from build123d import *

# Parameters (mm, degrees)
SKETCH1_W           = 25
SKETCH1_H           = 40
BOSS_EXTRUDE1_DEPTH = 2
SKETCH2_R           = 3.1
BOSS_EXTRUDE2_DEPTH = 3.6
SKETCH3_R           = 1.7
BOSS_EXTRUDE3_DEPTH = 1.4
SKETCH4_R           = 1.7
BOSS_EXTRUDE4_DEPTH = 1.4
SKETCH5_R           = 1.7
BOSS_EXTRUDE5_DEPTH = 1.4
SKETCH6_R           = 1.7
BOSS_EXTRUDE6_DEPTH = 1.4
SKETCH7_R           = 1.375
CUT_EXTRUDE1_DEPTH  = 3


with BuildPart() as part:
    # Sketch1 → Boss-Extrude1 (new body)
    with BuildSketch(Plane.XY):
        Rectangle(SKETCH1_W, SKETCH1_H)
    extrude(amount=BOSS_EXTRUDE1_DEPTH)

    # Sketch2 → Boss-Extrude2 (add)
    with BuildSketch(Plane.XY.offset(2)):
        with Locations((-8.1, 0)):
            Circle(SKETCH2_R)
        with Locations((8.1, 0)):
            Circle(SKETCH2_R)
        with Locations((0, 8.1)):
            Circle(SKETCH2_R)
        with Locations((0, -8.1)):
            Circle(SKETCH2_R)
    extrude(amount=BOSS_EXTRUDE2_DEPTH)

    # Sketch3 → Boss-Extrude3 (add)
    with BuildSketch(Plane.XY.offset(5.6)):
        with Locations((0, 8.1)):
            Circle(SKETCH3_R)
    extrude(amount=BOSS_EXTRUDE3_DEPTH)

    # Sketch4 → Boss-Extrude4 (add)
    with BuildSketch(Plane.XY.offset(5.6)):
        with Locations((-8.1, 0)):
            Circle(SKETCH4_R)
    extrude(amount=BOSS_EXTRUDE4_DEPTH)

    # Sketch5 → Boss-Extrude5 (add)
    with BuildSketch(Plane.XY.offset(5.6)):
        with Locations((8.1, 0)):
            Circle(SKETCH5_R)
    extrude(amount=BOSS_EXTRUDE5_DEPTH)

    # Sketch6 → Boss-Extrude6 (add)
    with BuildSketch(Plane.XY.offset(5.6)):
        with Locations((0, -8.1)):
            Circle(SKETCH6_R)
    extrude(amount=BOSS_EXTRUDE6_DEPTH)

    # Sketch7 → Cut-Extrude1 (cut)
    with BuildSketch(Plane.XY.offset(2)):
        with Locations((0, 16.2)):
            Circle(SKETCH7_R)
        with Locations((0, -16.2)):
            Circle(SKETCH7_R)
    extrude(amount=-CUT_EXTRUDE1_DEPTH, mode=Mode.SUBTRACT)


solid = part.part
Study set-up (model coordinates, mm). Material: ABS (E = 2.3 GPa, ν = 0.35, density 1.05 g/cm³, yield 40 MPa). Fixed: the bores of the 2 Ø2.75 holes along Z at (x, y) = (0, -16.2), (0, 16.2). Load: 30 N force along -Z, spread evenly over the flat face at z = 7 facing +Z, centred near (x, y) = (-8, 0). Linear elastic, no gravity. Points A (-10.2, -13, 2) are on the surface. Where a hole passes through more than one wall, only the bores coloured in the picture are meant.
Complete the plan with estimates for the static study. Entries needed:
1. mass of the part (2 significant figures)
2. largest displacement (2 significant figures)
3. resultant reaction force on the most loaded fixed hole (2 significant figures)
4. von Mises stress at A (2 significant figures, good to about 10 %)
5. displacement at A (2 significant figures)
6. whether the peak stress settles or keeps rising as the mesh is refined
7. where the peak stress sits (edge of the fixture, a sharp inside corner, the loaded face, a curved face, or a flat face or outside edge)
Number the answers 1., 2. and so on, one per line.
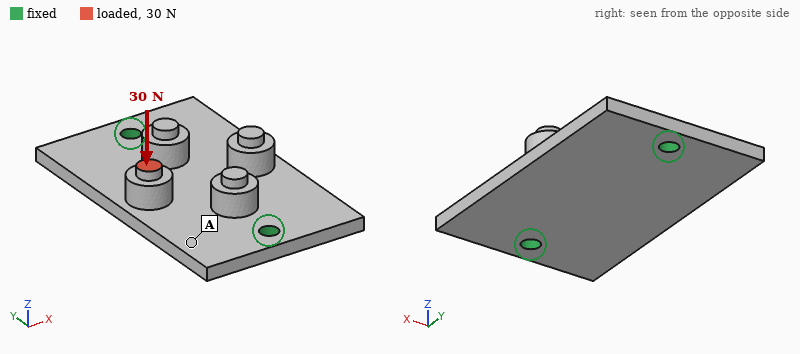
1. 2.6 g
2. 0.51 mm
3. 16 N
4. 3.5 MPa
5. 0.21 mm
6. keeps rising
7. edge of the fixture
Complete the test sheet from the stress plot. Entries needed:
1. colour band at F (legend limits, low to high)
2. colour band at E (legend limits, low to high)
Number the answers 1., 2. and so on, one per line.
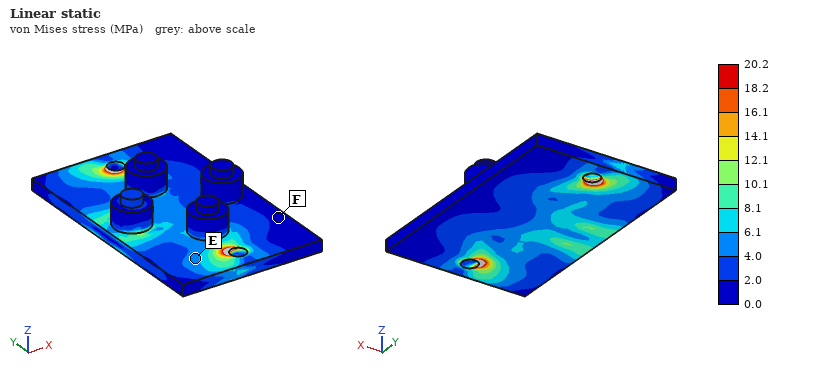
1. 0.0 to 2.0 MPa
2. 4.0 to 6.1 MPa
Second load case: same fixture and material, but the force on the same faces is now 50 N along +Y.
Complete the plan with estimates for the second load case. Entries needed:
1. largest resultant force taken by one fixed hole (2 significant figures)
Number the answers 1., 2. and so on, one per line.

1. 30 N
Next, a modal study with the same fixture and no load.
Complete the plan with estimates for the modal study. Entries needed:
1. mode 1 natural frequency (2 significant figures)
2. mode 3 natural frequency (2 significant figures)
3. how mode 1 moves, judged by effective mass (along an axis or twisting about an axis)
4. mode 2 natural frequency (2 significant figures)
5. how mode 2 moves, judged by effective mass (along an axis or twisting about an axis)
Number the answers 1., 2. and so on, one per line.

1. 1700 Hz
2. 3700 Hz
3. twisting about Y
4. 2000 Hz
5. along Z
